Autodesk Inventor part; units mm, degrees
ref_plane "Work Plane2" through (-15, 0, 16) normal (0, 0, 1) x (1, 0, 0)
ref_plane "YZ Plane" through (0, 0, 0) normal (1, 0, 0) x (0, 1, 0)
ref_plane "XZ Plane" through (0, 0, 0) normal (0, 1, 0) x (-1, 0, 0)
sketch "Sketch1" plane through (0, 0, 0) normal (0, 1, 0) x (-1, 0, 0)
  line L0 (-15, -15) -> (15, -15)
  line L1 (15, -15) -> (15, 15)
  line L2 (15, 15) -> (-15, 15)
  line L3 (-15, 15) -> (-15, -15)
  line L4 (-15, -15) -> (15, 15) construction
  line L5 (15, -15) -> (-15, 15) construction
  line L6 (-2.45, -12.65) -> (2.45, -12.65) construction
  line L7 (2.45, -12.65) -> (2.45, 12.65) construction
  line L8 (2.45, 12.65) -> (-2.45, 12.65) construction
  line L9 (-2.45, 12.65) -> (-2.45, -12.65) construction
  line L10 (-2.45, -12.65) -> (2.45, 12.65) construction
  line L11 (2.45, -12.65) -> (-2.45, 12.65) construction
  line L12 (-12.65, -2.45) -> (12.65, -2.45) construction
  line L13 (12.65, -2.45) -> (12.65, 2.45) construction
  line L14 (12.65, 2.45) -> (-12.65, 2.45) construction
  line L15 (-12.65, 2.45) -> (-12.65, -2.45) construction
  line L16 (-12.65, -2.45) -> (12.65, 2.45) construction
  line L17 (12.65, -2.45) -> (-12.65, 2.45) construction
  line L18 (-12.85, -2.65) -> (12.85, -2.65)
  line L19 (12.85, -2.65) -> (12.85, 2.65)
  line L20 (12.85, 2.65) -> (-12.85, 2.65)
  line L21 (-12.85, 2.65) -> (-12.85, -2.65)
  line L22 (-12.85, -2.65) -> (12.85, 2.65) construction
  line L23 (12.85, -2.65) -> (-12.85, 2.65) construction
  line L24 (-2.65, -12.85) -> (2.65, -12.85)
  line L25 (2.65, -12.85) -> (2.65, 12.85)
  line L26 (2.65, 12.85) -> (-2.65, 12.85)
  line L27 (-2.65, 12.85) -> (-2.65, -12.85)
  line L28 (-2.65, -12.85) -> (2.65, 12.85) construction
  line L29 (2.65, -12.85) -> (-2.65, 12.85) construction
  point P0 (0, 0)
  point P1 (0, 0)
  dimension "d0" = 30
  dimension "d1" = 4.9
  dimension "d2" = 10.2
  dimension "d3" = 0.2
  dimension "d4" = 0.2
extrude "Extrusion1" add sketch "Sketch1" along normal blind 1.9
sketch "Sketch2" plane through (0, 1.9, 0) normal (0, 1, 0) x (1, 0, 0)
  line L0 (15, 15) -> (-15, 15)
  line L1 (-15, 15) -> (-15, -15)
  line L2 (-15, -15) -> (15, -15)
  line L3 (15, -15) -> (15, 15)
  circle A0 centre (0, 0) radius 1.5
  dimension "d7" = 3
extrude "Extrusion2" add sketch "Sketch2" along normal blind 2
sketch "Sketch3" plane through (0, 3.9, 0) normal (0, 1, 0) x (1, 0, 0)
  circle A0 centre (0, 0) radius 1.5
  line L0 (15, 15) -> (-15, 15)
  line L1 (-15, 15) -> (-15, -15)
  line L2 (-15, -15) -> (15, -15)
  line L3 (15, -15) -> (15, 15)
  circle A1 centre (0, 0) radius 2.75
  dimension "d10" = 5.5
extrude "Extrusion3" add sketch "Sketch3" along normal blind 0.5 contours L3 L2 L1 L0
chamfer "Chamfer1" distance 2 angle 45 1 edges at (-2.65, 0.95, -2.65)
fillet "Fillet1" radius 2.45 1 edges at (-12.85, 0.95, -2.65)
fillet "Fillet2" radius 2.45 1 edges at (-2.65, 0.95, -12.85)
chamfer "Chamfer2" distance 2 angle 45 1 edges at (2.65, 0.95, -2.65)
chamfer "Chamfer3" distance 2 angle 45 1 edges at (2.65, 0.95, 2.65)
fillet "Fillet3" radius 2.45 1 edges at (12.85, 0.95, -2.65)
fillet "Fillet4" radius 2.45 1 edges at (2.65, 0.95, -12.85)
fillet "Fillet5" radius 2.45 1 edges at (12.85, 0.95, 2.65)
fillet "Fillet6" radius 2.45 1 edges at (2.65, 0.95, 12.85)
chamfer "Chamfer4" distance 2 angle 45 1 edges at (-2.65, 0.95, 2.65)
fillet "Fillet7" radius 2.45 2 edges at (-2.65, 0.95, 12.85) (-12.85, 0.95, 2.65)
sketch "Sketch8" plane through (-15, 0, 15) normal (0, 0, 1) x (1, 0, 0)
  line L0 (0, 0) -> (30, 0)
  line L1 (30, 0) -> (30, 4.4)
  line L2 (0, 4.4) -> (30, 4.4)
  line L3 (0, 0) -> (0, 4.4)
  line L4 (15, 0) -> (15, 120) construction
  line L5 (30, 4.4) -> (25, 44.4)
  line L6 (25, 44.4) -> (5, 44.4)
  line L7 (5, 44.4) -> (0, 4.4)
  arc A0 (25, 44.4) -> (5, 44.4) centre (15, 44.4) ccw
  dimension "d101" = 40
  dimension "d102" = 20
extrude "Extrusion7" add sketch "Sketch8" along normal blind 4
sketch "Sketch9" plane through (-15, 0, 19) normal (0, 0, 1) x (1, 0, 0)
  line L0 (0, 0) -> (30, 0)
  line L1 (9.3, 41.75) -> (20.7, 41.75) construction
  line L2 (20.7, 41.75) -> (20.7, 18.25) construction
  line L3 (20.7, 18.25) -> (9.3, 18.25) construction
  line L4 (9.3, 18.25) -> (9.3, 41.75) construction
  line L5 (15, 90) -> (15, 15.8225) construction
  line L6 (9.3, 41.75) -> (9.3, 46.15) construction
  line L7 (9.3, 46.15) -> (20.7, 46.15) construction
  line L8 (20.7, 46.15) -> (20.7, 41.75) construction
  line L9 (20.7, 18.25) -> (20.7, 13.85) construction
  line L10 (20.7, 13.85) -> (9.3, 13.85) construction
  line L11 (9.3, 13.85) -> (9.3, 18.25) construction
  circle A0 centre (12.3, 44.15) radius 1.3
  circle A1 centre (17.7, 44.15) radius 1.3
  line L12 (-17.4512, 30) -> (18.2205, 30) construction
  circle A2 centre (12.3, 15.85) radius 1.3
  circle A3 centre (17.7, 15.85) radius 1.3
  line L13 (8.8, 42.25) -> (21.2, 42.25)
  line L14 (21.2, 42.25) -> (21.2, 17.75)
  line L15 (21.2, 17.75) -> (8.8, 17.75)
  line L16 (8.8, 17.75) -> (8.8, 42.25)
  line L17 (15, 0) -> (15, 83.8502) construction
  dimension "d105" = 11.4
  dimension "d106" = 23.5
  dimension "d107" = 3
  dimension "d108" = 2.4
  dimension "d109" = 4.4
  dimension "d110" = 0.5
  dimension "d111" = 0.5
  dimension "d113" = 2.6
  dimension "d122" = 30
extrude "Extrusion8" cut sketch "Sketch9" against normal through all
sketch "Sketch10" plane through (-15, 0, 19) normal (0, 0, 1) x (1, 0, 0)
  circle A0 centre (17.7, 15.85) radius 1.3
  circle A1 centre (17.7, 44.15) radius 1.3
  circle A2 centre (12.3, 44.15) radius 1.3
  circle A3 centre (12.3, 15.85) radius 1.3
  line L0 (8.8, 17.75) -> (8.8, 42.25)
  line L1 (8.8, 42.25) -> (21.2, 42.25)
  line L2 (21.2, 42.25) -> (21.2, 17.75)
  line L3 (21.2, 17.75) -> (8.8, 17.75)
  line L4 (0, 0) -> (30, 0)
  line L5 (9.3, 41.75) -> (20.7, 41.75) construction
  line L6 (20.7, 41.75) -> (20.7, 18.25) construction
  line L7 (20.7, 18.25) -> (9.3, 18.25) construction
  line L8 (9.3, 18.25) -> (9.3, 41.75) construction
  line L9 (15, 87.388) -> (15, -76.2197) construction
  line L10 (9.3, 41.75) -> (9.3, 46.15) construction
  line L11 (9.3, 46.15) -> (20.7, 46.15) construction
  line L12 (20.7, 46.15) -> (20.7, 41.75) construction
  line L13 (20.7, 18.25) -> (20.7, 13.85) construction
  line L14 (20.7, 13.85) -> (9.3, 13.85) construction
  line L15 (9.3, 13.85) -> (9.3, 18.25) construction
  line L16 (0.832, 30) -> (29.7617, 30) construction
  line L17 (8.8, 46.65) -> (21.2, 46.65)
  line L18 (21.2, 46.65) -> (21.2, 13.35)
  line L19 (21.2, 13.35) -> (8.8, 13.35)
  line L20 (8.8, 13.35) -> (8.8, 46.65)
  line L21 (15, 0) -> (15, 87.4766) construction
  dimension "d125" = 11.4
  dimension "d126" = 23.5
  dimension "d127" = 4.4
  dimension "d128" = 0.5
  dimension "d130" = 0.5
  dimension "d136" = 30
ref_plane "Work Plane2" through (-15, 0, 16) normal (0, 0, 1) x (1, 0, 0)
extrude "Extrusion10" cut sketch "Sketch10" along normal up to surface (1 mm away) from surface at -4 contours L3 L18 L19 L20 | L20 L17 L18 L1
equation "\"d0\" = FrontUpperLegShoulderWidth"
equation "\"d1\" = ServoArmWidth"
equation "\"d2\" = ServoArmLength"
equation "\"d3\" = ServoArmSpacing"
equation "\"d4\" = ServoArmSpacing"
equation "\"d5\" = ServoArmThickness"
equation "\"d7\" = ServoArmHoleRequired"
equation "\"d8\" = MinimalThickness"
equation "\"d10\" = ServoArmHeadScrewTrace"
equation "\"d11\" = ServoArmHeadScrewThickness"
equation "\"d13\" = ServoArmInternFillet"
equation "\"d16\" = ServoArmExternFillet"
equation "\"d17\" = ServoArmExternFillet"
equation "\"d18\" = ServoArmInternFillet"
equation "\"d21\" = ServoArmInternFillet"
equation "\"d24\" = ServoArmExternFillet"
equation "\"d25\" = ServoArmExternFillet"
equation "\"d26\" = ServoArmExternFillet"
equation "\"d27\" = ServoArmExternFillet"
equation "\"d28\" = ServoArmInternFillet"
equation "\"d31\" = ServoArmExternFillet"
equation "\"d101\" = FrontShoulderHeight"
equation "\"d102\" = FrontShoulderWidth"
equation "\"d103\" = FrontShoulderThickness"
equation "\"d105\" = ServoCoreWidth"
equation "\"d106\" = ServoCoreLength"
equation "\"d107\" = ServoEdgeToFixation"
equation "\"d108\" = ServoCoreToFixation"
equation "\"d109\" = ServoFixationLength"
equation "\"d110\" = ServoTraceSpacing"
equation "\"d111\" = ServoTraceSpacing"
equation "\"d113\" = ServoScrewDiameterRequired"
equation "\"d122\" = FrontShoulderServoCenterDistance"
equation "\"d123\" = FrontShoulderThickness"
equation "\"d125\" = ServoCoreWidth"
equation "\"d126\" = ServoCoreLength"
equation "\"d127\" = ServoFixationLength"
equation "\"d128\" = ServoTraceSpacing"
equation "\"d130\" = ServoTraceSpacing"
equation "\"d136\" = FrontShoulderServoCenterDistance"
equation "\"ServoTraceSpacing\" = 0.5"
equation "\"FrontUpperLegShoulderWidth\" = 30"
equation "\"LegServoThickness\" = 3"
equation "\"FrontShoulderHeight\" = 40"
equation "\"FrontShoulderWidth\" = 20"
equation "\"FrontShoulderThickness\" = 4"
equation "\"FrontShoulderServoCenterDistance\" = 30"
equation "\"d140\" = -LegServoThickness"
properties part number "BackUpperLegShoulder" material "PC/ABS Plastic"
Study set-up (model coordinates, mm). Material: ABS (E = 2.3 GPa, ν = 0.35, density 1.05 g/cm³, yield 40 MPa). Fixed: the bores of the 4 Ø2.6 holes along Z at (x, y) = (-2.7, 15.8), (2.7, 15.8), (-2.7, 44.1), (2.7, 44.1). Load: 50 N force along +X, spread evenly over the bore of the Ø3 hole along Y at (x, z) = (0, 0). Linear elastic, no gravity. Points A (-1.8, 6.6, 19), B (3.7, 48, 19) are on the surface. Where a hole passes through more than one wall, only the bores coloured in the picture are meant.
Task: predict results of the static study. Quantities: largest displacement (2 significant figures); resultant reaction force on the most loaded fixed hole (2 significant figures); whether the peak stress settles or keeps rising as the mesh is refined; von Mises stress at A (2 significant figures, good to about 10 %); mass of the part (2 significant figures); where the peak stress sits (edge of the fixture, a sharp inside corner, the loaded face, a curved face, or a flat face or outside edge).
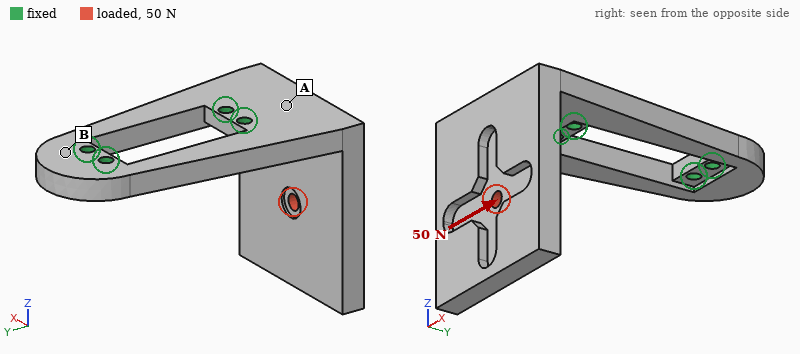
0.84 mm
97 N
keeps rising
6.2 MPa
7.6 g
edge of the fixture
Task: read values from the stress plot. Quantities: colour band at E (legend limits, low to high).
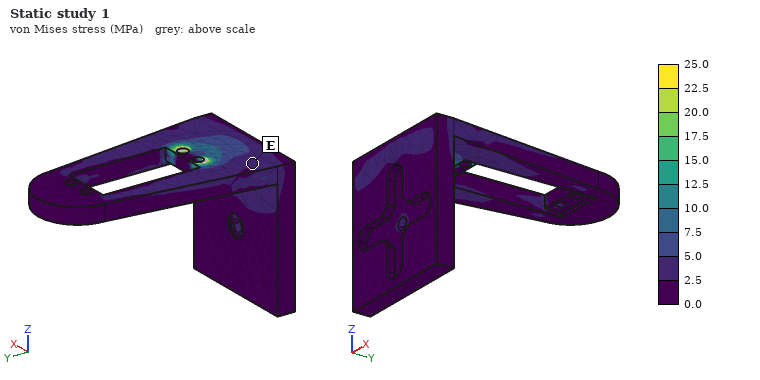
2.5 to 5.0 MPa
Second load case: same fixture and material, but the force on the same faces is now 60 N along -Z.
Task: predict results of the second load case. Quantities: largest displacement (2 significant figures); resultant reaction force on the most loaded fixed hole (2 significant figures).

0.77 mm
35 N
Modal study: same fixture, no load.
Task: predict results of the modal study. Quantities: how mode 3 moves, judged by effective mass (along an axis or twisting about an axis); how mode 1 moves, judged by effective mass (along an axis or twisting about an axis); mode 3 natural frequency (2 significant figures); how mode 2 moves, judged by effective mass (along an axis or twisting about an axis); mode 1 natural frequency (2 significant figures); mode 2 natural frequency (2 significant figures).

along Z
along Y
1700 Hz
along X
500 Hz
730 Hz
